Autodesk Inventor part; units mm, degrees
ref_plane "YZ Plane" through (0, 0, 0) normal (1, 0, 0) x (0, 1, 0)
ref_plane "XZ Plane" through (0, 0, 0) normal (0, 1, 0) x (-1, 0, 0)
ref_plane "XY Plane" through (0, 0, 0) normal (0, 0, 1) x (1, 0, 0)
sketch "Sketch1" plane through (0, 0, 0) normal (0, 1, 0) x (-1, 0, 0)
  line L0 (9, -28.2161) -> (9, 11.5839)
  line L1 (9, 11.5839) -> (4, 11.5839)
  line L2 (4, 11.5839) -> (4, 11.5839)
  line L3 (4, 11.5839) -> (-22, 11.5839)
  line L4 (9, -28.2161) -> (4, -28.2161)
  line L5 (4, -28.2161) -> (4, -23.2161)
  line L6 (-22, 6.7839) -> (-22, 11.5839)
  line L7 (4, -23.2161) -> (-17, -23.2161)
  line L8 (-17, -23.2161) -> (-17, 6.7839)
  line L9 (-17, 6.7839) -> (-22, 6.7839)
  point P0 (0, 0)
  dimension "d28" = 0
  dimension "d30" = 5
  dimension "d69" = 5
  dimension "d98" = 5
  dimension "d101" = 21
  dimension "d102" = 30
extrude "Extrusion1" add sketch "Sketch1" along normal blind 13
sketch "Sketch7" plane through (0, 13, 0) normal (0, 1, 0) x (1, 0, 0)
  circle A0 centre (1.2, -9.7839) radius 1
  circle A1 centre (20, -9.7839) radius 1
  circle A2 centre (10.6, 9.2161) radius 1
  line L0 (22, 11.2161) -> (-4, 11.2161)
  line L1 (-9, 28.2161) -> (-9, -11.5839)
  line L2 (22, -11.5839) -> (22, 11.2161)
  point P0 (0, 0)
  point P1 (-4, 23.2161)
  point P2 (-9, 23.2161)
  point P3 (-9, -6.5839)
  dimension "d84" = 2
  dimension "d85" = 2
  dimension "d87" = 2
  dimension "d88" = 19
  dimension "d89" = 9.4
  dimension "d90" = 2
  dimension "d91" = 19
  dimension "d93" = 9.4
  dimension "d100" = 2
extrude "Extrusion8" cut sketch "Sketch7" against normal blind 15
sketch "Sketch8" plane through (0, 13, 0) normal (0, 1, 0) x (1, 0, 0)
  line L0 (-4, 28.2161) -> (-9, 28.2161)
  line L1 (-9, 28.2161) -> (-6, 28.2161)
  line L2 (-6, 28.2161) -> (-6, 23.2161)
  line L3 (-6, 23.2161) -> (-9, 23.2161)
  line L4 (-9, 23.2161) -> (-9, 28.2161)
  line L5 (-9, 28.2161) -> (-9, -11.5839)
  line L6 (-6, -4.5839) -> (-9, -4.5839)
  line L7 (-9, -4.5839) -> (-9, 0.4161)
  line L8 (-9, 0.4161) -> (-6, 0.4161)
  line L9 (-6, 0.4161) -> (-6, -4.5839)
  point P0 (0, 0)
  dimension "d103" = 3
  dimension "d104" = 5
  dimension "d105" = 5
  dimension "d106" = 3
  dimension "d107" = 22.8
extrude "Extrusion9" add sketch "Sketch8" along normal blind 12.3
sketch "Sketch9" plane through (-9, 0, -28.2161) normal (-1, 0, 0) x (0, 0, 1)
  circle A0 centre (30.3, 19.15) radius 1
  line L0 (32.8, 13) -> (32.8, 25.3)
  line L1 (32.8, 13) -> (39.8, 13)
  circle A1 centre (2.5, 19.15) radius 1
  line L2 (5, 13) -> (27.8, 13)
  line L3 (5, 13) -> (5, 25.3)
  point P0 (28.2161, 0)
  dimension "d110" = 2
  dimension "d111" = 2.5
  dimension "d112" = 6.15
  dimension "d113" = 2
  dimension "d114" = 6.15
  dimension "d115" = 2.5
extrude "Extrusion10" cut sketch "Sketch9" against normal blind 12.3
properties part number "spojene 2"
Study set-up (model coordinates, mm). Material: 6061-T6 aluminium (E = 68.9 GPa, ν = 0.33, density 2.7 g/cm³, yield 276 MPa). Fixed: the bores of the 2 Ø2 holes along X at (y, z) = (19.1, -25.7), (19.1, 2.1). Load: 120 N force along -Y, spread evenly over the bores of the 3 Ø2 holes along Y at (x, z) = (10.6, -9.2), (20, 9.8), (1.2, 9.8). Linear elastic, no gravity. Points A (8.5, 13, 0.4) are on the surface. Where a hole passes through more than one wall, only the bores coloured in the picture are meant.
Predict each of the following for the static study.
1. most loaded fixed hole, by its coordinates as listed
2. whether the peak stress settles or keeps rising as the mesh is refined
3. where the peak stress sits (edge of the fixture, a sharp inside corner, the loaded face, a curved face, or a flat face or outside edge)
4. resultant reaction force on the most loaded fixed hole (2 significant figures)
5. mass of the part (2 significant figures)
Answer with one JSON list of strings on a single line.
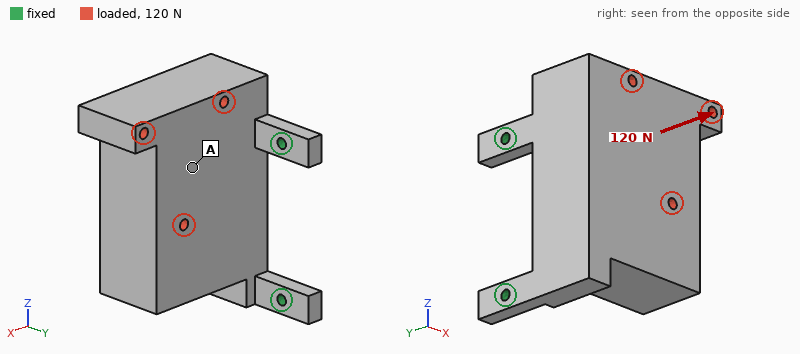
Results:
["(19.1, 2.1)", "keeps rising", "edge of the fixture", "120 N", "34 g"]
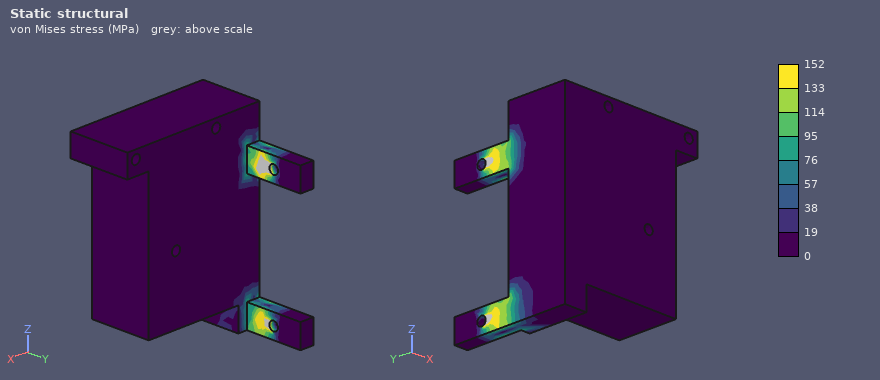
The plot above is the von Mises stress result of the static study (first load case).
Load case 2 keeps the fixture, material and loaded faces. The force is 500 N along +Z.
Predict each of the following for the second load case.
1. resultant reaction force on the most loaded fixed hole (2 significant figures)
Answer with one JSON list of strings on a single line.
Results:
["440 N"]
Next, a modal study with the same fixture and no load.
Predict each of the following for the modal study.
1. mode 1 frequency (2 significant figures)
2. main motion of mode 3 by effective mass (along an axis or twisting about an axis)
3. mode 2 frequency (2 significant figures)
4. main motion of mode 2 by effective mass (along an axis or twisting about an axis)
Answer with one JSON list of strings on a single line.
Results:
["770 Hz", "along X", "3400 Hz", "along Z"]
